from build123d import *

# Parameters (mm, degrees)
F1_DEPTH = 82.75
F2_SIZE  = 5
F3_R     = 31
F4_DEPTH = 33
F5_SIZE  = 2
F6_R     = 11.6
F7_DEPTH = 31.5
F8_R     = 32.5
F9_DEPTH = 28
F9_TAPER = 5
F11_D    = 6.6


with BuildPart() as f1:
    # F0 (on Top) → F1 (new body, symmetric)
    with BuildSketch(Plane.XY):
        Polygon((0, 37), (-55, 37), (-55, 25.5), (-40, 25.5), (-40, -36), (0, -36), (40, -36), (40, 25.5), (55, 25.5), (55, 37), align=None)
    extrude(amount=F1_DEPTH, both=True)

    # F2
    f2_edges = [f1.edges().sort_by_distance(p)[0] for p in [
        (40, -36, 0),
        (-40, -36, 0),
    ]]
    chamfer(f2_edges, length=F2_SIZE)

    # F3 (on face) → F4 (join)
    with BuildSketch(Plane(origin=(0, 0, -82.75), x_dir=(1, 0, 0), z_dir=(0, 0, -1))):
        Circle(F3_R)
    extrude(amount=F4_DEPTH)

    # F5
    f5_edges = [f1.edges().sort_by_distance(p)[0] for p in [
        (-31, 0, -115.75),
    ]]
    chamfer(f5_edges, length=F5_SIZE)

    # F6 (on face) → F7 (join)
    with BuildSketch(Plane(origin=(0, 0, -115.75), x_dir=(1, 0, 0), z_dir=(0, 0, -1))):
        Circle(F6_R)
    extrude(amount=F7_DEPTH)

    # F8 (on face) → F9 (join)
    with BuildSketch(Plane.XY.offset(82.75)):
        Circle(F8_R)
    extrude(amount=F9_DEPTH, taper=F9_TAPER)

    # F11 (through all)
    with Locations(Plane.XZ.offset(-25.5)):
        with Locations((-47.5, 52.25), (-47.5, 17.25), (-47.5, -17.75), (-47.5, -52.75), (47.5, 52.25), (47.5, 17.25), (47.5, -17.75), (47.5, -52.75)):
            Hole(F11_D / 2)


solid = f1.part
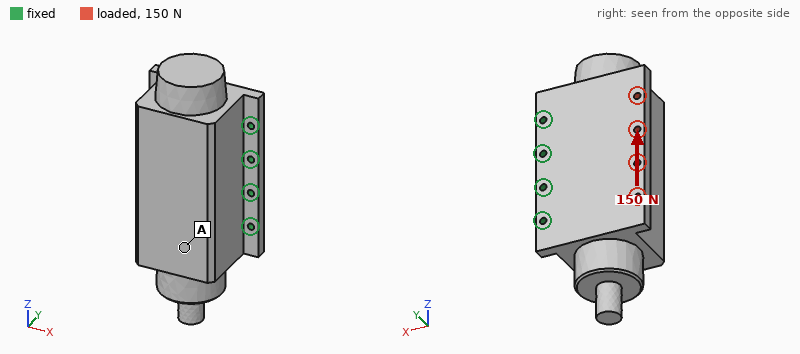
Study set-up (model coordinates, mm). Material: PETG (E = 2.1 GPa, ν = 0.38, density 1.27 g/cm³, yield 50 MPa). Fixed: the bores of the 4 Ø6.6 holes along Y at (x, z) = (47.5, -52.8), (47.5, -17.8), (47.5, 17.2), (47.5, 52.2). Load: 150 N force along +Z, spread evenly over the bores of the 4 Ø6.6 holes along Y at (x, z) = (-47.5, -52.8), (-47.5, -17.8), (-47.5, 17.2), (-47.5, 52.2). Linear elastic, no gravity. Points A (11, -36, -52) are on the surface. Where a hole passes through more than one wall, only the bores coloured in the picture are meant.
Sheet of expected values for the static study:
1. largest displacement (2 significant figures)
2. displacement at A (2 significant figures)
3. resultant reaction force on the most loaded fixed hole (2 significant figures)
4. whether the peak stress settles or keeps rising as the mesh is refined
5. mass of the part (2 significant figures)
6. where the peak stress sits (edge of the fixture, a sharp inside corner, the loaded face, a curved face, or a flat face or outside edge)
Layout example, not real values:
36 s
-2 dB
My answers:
25 µm
8.8 µm
120 N
keeps rising
1.5 kg
edge of the fixture
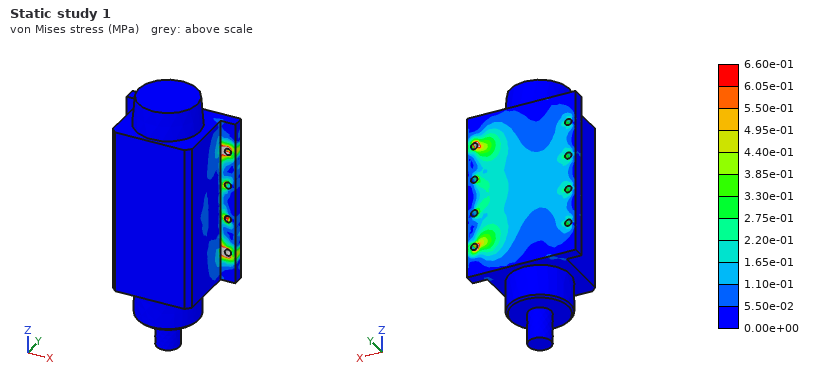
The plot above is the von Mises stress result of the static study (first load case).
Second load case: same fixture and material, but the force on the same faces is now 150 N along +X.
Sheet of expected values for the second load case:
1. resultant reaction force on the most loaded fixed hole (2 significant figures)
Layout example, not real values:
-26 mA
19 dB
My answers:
39 N
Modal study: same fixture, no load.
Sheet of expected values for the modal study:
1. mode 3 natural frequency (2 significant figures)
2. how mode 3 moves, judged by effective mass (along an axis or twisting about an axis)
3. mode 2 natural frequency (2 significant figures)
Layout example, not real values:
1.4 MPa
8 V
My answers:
540 Hz
along Z
420 Hz
